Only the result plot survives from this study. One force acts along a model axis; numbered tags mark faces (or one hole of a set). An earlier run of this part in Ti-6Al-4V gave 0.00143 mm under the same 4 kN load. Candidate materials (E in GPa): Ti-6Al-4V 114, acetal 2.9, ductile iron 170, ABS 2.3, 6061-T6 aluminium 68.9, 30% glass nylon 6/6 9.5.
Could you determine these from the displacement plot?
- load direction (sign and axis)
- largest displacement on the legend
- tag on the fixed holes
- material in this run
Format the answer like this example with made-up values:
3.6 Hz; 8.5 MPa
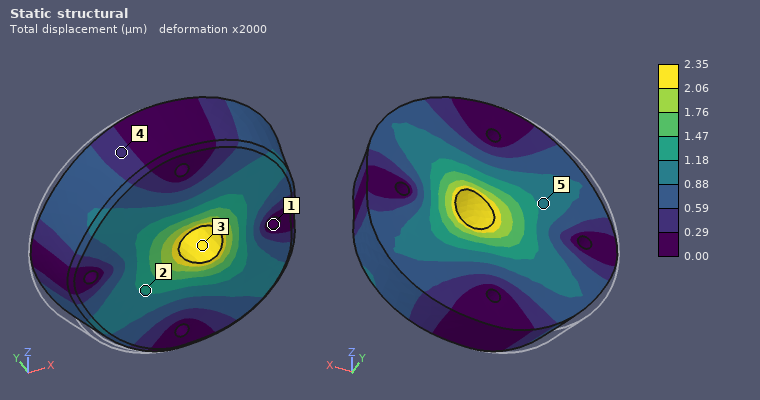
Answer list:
+X; 2.35 µm; 1; 6061-T6 aluminium
